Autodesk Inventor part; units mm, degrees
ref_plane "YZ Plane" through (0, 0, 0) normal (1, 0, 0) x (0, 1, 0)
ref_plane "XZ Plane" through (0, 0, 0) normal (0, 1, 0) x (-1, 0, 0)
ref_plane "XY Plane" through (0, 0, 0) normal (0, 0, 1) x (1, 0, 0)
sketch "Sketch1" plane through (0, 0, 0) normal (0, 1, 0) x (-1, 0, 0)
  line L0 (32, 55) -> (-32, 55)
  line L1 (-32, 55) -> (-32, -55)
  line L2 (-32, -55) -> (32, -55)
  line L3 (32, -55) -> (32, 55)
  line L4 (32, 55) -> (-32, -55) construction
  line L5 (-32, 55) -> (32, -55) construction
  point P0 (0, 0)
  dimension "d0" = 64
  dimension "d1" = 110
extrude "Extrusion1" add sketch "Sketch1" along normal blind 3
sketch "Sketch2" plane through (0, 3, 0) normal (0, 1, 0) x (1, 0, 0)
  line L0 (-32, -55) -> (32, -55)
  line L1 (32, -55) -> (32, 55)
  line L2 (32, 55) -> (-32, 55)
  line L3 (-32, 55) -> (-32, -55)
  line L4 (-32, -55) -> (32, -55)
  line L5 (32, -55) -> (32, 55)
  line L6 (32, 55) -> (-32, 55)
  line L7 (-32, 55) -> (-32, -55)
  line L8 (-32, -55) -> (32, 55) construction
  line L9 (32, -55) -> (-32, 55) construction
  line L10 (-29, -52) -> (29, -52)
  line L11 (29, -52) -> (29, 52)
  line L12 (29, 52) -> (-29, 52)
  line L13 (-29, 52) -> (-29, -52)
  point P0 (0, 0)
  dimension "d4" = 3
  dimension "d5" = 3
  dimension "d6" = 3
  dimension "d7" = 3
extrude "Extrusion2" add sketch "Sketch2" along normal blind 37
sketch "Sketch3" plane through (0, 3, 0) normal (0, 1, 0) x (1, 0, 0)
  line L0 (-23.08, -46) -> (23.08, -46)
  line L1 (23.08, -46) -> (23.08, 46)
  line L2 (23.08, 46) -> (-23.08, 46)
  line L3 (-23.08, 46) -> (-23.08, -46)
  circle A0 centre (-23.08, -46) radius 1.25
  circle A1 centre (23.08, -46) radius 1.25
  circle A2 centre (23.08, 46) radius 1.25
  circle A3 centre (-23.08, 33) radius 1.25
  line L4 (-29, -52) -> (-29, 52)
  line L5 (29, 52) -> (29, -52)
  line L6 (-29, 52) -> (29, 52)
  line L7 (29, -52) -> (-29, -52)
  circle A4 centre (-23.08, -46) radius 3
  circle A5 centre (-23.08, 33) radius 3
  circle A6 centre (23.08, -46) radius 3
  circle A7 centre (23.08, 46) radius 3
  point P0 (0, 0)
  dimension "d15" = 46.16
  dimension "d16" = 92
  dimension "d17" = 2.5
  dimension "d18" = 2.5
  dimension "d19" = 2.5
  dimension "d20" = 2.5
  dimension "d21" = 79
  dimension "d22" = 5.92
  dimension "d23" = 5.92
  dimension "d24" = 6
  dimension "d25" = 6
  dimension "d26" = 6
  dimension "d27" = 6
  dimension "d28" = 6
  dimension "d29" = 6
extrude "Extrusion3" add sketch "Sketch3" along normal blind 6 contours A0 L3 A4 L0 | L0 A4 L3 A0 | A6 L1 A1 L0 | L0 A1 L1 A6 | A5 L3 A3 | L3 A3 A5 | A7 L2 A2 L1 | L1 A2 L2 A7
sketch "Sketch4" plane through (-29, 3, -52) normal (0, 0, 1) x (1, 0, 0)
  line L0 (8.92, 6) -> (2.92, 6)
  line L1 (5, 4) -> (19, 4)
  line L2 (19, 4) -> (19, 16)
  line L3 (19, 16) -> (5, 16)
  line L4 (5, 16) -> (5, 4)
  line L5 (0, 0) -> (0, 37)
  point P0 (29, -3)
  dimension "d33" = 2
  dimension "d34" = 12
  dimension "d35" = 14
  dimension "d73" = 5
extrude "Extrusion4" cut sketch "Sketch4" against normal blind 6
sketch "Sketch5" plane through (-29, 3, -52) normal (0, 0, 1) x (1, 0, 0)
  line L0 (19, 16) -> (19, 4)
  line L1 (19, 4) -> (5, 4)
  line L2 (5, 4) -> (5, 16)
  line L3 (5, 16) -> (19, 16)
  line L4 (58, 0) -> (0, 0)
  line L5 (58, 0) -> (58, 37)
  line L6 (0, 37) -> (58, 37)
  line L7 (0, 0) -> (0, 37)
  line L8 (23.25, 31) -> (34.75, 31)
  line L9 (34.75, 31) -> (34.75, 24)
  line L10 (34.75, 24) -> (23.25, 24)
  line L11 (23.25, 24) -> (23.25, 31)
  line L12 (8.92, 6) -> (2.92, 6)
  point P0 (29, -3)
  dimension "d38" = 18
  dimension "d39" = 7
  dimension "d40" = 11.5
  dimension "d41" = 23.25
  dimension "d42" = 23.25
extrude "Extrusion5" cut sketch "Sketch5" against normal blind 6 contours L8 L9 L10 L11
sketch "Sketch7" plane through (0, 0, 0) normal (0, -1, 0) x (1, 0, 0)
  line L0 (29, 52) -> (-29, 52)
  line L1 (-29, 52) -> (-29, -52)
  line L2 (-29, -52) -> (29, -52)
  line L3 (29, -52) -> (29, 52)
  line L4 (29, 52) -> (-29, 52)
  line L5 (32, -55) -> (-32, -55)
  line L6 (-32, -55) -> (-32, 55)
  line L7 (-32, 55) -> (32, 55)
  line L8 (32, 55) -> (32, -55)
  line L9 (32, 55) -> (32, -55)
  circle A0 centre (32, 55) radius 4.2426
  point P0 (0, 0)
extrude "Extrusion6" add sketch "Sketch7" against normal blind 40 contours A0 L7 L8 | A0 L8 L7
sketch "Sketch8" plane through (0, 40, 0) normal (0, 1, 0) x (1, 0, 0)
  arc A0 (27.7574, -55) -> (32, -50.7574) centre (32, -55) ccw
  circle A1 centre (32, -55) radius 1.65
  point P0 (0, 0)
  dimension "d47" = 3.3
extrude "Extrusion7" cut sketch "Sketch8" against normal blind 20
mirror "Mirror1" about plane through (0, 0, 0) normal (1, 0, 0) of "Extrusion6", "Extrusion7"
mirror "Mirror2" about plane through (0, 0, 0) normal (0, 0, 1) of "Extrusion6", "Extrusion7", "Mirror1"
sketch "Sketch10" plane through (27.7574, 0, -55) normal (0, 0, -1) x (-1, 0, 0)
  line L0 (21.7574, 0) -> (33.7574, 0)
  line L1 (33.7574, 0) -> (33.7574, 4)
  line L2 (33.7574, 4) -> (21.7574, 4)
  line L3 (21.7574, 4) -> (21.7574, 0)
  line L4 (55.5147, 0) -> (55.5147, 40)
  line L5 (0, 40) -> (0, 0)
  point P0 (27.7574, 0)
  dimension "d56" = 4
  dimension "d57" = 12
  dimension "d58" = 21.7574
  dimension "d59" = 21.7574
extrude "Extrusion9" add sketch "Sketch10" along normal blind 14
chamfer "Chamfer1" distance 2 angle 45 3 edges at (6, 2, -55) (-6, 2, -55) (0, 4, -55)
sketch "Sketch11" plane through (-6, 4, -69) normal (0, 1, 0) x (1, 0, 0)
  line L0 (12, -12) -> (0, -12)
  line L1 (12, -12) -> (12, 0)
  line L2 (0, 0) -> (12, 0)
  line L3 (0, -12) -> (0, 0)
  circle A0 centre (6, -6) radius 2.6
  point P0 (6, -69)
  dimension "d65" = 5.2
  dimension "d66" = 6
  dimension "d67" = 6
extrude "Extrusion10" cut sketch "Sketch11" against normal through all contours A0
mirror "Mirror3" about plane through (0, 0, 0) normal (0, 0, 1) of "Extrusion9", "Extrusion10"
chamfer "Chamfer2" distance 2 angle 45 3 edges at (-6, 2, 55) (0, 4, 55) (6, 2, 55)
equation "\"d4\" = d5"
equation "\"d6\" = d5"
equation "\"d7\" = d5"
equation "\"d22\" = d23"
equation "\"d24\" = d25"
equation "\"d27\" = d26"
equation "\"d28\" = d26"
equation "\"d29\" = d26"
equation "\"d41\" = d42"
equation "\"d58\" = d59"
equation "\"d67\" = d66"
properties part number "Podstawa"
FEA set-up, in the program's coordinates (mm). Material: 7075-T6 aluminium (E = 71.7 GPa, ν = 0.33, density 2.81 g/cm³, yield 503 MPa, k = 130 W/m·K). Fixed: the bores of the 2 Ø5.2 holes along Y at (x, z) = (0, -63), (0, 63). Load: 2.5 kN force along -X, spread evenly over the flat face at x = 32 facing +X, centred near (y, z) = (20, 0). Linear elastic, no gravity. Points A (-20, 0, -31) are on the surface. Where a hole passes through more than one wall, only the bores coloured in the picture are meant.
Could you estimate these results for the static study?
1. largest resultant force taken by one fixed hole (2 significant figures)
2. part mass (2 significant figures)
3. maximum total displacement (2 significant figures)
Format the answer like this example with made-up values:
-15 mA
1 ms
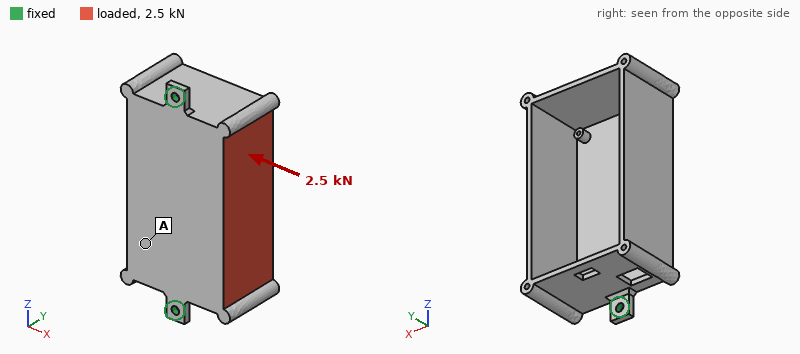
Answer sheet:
1.3 kN
180 g
1.6 mm
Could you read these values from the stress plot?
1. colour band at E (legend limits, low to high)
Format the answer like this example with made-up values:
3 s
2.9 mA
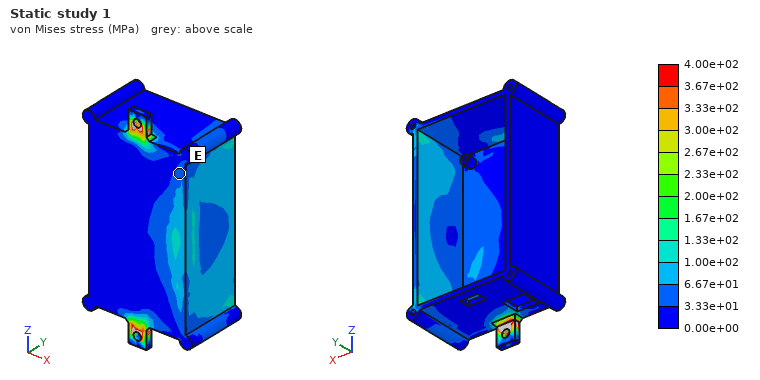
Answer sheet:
3.33e+01 to 6.67e+01 MPa
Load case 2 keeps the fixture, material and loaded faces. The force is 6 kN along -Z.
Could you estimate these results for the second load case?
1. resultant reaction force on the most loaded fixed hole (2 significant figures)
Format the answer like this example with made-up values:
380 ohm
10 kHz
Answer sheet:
3.5 kN
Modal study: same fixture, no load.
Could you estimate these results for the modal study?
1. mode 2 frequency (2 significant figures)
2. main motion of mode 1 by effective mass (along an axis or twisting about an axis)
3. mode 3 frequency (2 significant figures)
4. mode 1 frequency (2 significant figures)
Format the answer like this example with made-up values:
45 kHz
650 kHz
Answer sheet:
1100 Hz
along X
2000 Hz
590 Hz
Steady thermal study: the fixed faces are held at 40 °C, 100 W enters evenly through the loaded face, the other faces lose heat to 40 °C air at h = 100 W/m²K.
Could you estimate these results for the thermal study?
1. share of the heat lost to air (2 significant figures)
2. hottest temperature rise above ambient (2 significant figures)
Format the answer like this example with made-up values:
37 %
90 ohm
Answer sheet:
81 %
66 K
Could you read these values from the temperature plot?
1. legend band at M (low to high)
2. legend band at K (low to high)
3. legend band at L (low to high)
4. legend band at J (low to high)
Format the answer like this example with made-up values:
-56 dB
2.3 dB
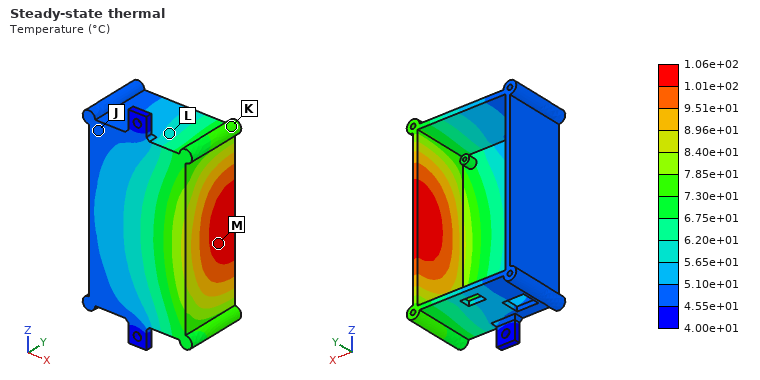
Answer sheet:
1.01e+02 to 1.06e+02 °C
7.30e+01 to 7.85e+01 °C
5.65e+01 to 6.20e+01 °C
4.55e+01 to 5.10e+01 °C
